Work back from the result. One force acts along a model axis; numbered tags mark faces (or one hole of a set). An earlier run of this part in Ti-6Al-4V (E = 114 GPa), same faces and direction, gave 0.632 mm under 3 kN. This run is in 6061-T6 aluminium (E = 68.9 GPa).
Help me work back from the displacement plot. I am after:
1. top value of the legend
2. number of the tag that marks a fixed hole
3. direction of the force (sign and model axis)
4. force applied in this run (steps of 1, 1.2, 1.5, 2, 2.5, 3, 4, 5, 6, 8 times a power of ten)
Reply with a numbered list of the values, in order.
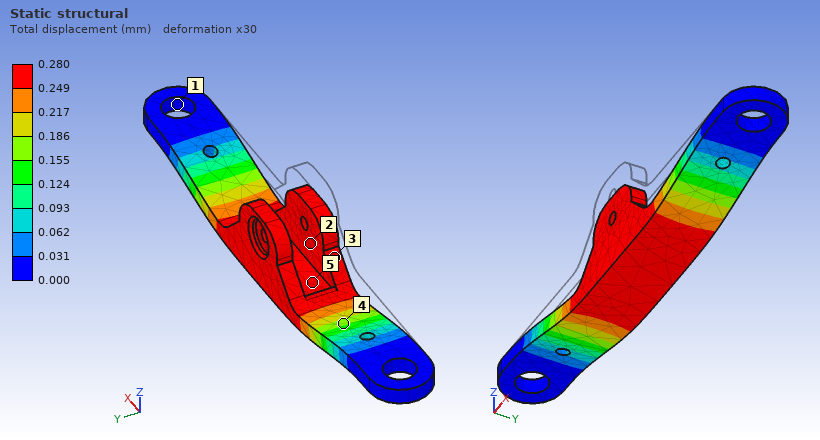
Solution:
1. 0.280 mm
2. 1
3. -Z
4. 800 N
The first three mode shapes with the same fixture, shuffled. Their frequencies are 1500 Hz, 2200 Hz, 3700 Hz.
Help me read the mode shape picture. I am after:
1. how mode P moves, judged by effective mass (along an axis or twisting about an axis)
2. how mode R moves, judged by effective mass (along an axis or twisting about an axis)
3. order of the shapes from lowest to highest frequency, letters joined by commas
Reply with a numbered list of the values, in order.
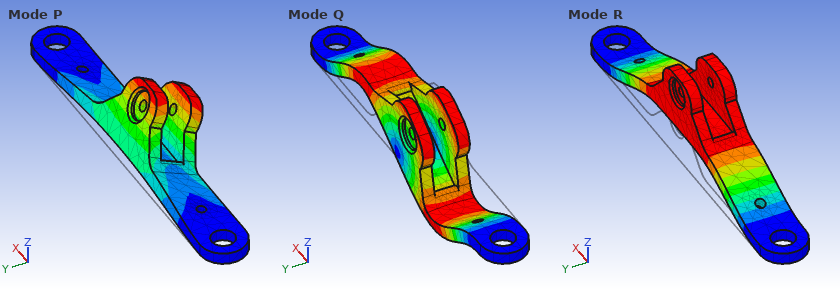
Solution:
1. along Y
2. along Z
3. R, P, Q
